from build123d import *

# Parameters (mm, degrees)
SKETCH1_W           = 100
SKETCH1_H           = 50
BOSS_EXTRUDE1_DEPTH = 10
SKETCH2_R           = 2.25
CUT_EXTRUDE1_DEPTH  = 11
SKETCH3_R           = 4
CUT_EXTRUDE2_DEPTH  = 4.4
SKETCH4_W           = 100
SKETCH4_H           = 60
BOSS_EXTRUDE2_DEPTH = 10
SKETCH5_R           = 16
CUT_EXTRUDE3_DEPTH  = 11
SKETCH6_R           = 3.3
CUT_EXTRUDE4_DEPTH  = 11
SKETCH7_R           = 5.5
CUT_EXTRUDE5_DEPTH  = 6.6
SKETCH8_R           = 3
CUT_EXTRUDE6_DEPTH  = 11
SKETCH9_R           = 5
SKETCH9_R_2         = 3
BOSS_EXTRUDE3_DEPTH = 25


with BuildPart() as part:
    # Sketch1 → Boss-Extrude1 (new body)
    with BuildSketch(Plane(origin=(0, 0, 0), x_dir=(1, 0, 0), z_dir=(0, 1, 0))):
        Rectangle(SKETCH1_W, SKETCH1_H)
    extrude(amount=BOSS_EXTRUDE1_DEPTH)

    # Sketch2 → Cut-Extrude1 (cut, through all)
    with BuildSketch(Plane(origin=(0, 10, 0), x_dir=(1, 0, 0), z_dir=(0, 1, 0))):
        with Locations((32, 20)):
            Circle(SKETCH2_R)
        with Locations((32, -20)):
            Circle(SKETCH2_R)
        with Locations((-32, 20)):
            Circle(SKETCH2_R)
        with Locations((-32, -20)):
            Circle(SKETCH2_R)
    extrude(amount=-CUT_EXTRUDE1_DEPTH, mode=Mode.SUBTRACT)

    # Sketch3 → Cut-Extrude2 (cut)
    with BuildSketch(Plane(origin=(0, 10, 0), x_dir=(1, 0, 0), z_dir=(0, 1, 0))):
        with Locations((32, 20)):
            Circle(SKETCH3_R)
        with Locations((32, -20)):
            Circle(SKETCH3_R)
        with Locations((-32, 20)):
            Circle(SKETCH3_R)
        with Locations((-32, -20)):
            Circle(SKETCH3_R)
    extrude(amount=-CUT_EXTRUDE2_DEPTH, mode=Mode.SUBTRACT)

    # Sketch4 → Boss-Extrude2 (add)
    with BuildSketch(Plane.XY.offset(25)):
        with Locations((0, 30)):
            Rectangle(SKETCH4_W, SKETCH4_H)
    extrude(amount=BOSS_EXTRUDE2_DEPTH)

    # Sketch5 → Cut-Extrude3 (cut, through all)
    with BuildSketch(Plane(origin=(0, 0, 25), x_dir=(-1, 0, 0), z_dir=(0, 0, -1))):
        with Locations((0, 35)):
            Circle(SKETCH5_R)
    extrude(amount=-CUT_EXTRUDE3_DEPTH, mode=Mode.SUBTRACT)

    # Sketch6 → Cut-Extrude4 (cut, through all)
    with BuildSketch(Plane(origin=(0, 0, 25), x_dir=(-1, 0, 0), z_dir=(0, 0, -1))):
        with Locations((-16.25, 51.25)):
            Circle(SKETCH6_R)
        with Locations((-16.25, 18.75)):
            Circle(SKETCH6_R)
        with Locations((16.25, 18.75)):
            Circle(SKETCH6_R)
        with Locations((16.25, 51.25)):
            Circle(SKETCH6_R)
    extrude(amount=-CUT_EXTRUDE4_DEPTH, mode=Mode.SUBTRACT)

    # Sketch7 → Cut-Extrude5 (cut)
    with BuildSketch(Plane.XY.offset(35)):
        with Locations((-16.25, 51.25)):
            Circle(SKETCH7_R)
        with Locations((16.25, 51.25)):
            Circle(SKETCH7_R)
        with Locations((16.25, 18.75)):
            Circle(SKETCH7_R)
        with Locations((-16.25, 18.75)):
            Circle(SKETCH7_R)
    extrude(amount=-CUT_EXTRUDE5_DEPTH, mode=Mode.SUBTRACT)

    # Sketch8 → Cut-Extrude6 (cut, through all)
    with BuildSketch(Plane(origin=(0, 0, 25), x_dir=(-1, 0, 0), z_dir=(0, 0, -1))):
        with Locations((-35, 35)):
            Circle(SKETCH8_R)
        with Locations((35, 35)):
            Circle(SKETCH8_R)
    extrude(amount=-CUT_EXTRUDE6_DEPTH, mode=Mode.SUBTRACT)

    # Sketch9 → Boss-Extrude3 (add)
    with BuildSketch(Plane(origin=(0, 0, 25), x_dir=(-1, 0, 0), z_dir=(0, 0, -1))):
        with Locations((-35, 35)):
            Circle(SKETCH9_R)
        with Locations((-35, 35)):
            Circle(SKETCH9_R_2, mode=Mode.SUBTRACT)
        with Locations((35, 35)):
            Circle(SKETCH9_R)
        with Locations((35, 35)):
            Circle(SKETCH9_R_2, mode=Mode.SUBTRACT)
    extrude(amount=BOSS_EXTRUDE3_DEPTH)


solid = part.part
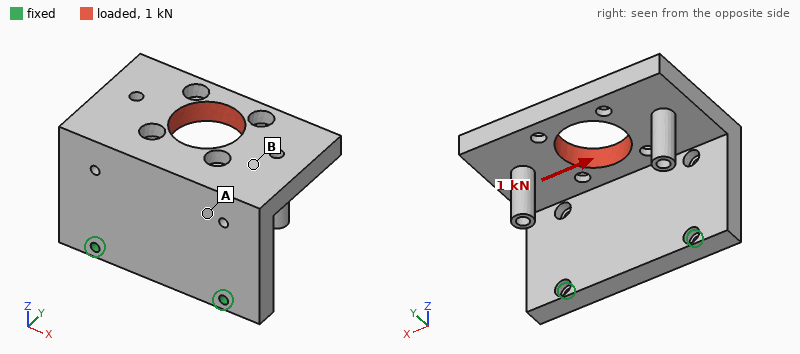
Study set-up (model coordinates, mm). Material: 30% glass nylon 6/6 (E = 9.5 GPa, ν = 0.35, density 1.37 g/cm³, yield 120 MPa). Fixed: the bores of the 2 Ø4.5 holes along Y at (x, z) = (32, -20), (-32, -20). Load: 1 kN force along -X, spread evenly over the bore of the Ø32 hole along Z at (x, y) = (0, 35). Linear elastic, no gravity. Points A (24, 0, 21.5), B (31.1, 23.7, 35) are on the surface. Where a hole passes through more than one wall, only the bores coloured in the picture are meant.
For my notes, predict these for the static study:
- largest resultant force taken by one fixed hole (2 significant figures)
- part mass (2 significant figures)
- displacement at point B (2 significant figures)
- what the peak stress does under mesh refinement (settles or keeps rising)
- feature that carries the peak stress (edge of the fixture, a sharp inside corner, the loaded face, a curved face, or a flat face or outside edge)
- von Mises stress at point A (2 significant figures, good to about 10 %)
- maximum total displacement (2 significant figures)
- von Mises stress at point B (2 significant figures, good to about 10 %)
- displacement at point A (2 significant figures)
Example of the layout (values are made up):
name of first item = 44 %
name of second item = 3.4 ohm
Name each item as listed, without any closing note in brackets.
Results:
largest resultant force taken by one fixed hole = 1.0 kN
part mass = 140 g
displacement at point B = 0.32 mm
what the peak stress does under mesh refinement = keeps rising
feature that carries the peak stress = edge of the fixture
von Mises stress at point A = 8.1 MPa
maximum total displacement = 0.68 mm
von Mises stress at point B = 3.0 MPa
displacement at point A = 0.17 mm
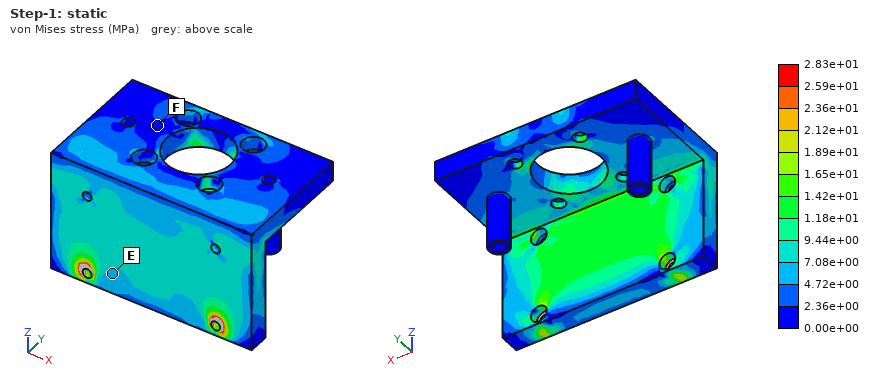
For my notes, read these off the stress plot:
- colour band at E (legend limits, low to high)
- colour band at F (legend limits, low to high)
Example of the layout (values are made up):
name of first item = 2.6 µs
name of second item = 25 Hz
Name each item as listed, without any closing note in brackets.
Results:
colour band at E = 4.72e+00 to 7.08e+00 MPa
colour band at F = 0.00e+00 to 2.36e+00 MPa
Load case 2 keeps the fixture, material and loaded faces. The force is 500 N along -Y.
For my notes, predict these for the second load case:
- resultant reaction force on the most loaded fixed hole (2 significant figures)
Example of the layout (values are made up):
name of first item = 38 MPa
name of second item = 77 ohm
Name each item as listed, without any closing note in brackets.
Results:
resultant reaction force on the most loaded fixed hole = 250 N
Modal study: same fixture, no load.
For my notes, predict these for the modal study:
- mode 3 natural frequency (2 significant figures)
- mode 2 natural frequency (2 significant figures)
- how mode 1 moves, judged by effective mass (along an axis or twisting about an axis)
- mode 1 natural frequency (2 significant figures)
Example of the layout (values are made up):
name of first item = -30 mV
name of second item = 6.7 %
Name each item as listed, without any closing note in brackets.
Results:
mode 3 natural frequency = 1100 Hz
mode 2 natural frequency = 750 Hz
how mode 1 moves, judged by effective mass = along Y
mode 1 natural frequency = 340 Hz
